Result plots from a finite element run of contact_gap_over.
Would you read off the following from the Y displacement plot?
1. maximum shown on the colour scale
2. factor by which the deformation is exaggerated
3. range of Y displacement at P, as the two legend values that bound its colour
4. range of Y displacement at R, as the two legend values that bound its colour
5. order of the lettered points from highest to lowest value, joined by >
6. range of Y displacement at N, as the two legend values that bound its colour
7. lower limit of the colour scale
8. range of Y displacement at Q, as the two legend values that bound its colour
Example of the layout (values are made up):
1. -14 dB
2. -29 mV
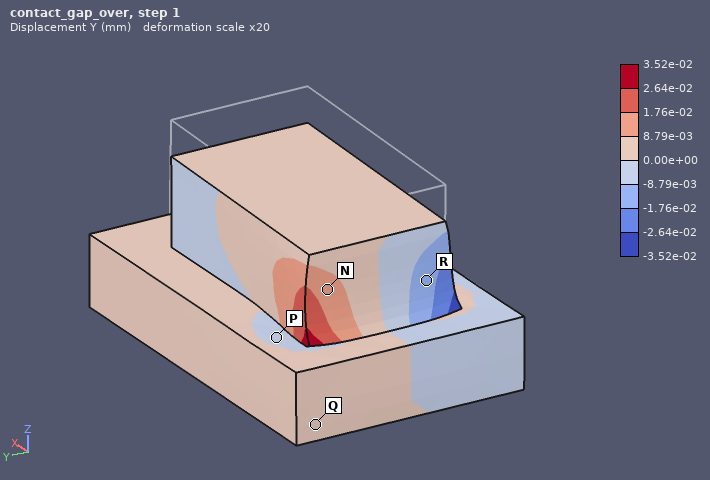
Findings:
1. 3.52e-02 mm
2. 20
3. -8.79e-03 to 0.00e+00 mm
4. -1.76e-02 to -8.79e-03 mm
5. N > Q > P > R
6. 8.79e-03 to 1.76e-02 mm
7. -3.52e-02 mm
8. 0.00e+00 to 8.79e-03 mm
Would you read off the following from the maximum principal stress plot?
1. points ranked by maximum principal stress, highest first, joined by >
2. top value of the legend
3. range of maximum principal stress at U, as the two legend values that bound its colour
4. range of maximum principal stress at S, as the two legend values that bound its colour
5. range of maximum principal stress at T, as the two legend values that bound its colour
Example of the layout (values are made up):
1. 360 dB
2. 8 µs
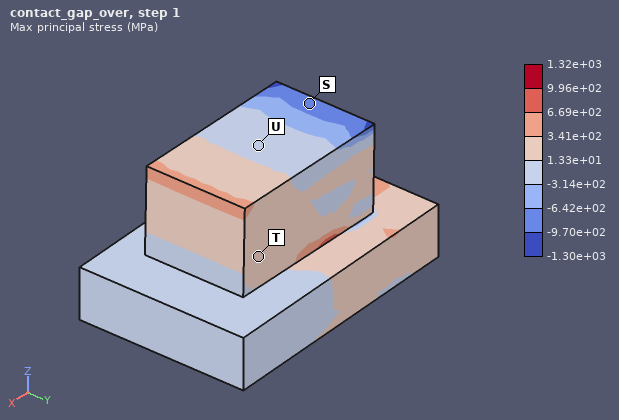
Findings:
1. T > U > S
2. 1.32e+03 MPa
3. -3.14e+02 to 1.33e+01 MPa
4. -9.70e+02 to -6.42e+02 MPa
5. 1.33e+01 to 3.41e+02 MPa
